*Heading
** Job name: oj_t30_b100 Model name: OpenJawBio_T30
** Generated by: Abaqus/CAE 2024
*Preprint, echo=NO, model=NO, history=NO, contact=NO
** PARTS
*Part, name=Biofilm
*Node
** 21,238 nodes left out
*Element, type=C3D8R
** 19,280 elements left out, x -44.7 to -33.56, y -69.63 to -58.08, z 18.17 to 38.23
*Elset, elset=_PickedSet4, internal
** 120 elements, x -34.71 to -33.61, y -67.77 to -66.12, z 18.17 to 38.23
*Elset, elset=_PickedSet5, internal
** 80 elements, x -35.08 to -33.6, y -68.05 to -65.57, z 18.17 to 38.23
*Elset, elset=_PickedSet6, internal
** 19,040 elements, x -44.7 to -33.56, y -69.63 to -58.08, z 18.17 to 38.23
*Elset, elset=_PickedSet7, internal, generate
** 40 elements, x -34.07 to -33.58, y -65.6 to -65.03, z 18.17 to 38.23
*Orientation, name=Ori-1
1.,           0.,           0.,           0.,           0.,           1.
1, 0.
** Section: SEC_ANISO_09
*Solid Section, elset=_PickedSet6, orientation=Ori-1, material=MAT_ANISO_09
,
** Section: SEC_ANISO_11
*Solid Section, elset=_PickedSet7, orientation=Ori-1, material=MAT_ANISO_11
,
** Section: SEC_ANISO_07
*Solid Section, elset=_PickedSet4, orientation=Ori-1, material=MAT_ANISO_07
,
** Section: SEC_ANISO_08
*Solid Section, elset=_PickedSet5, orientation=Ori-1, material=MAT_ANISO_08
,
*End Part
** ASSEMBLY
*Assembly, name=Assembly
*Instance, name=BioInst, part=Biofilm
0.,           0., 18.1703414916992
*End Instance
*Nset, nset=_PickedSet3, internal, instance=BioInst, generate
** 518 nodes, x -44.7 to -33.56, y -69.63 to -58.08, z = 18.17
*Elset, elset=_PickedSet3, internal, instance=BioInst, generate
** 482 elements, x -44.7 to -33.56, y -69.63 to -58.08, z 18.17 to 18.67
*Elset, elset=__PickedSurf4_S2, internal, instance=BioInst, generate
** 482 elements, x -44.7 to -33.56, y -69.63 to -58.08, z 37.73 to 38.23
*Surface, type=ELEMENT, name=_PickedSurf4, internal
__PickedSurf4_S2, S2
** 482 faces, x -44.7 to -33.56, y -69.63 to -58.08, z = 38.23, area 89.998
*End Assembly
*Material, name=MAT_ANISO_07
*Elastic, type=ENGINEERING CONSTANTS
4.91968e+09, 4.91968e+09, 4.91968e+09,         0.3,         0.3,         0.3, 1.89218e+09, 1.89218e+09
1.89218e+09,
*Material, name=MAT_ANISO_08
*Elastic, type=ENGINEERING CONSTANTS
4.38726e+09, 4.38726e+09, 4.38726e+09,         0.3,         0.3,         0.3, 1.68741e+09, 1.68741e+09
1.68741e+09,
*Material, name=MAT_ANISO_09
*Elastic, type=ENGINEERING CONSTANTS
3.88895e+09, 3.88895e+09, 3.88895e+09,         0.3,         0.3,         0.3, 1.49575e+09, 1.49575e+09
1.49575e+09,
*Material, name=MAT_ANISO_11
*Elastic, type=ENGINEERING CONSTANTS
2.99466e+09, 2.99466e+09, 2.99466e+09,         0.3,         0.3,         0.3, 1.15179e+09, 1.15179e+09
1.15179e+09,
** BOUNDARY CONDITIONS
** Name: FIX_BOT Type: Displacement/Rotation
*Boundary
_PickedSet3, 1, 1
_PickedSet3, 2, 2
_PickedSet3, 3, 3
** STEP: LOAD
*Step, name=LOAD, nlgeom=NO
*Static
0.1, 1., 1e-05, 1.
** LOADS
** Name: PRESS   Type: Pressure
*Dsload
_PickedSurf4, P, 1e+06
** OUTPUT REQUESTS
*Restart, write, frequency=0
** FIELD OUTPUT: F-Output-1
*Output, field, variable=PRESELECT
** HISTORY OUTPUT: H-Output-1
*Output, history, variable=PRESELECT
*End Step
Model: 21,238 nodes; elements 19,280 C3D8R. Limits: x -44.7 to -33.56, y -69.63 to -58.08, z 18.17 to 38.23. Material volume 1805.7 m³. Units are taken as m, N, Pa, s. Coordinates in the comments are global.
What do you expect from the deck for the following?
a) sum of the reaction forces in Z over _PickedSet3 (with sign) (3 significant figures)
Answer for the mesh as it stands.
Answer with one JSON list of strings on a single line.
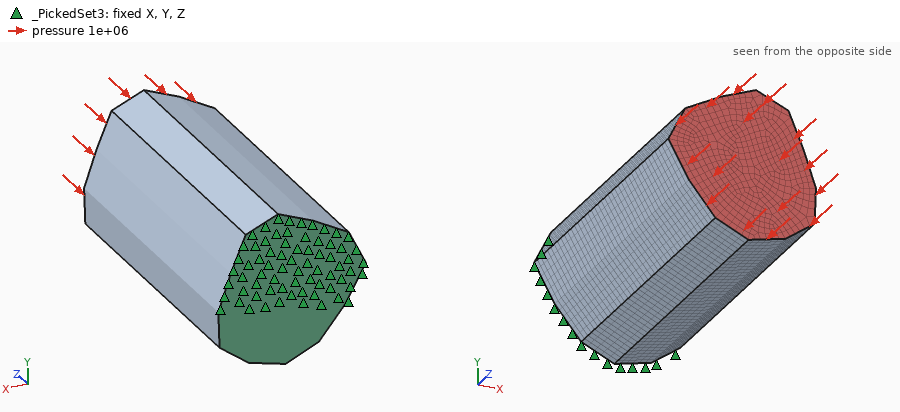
["9.00e+07 N"]
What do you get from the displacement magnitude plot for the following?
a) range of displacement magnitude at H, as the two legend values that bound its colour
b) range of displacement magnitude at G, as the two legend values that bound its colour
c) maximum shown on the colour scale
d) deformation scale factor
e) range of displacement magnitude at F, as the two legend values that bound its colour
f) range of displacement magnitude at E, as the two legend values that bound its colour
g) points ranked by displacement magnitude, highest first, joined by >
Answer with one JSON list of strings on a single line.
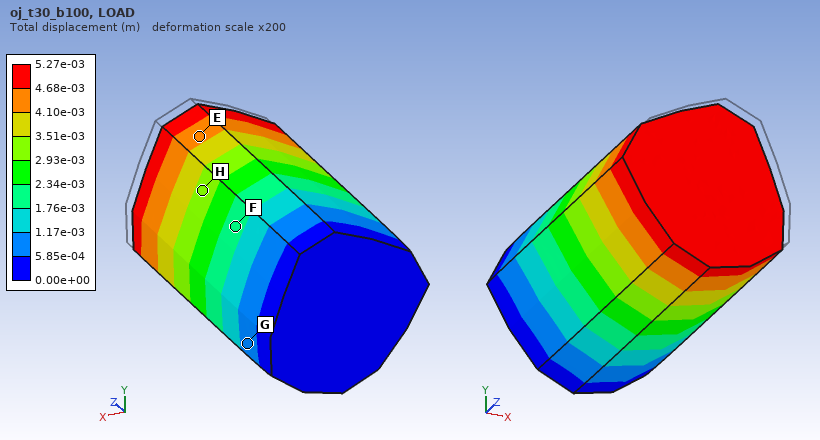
["2.93e-03 to 3.51e-03 m", "5.85e-04 to 1.17e-03 m", "5.27e-03 m", "200", "1.76e-03 to 2.34e-03 m", "4.10e-03 to 4.68e-03 m", "E > H > F > G"]
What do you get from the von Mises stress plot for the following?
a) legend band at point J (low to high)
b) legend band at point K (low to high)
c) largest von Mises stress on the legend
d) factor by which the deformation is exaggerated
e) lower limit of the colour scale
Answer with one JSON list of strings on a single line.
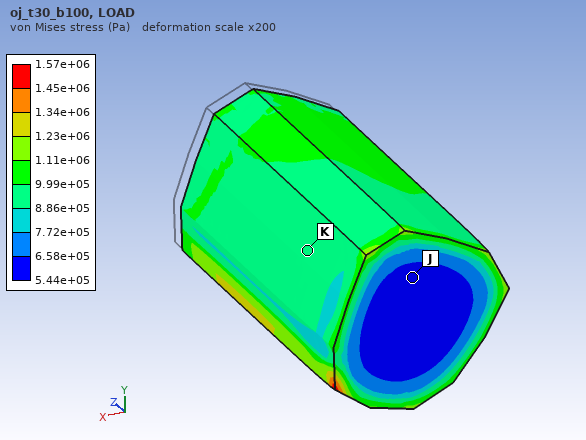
["5.44e+05 to 6.58e+05 Pa", "8.86e+05 to 9.99e+05 Pa", "1.57e+06 Pa", "200", "5.44e+05 Pa"]
